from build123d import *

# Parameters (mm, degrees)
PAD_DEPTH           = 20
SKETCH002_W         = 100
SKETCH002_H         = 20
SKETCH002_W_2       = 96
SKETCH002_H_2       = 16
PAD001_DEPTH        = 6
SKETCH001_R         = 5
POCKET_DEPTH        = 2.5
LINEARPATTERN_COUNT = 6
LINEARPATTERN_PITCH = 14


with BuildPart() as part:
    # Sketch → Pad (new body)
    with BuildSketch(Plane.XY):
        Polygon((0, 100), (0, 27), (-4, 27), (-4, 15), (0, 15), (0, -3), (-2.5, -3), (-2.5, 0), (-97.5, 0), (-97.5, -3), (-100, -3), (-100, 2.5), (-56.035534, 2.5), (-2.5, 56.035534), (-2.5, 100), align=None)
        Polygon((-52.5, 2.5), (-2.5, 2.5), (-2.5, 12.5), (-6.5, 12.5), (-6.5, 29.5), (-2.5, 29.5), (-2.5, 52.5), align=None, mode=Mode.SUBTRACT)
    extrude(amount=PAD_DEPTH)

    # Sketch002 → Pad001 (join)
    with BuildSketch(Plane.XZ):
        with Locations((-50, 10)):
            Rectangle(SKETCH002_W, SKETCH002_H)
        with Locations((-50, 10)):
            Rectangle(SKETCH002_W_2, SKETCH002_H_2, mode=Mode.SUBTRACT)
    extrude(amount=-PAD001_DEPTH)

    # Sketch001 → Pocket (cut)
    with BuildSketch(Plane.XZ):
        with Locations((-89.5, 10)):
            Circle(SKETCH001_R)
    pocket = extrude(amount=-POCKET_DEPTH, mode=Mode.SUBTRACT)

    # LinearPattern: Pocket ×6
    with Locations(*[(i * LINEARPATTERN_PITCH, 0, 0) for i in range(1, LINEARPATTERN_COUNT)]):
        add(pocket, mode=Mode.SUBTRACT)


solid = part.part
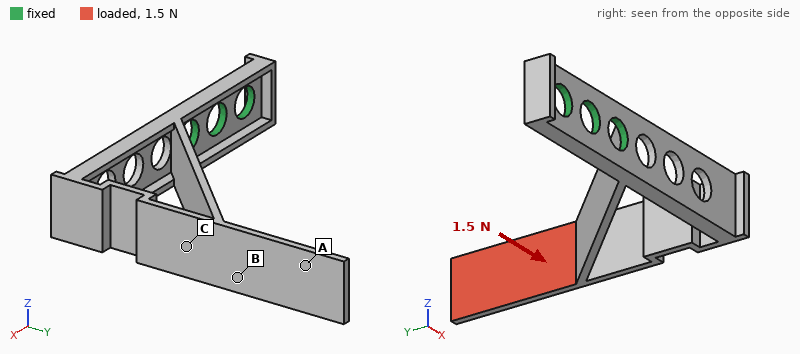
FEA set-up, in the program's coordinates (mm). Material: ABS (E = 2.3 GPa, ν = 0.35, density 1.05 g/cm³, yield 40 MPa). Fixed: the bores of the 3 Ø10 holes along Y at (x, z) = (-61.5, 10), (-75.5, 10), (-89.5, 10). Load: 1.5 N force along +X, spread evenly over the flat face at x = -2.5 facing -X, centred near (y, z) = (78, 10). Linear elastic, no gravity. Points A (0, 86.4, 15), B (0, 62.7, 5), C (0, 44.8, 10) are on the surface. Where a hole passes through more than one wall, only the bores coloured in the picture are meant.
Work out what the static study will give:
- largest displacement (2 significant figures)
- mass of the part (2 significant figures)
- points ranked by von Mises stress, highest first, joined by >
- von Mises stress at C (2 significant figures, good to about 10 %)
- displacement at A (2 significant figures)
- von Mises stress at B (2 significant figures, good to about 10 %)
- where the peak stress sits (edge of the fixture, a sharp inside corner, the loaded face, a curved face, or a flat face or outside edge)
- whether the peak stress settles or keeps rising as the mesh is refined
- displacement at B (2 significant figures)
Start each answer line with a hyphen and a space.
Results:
- 1.3 mm
- 15 g
- B > C > A
- 0.83 MPa
- 1.1 mm
- 1.1 MPa
- edge of the fixture
- keeps rising
- 0.70 mm
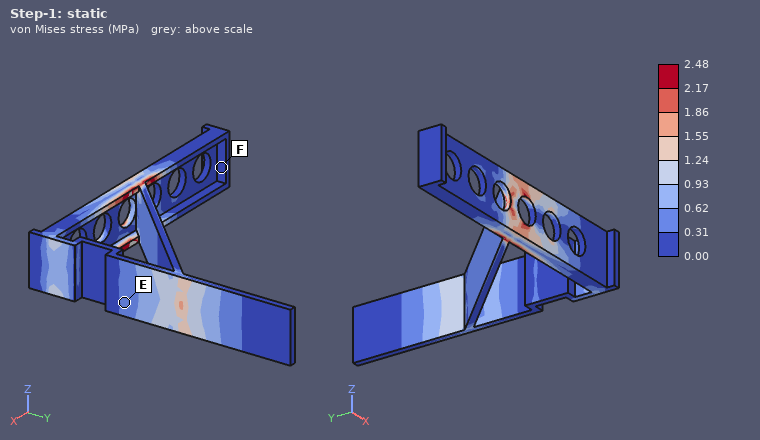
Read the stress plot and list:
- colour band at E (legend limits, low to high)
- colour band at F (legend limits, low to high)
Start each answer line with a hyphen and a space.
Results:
- 0.31 to 0.62 MPa
- 0.00 to 0.31 MPa
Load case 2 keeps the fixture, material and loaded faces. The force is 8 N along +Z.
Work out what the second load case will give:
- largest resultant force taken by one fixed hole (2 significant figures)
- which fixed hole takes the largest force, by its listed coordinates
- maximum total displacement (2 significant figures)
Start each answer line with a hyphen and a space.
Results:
- 13 N
- (-61.5, 10)
- 1.5 mm
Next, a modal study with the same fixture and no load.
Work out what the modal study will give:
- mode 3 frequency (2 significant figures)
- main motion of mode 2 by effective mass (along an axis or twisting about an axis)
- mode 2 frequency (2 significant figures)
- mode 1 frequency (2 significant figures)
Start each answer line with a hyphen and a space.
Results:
- 260 Hz
- along Z
- 230 Hz
- 92 Hz
